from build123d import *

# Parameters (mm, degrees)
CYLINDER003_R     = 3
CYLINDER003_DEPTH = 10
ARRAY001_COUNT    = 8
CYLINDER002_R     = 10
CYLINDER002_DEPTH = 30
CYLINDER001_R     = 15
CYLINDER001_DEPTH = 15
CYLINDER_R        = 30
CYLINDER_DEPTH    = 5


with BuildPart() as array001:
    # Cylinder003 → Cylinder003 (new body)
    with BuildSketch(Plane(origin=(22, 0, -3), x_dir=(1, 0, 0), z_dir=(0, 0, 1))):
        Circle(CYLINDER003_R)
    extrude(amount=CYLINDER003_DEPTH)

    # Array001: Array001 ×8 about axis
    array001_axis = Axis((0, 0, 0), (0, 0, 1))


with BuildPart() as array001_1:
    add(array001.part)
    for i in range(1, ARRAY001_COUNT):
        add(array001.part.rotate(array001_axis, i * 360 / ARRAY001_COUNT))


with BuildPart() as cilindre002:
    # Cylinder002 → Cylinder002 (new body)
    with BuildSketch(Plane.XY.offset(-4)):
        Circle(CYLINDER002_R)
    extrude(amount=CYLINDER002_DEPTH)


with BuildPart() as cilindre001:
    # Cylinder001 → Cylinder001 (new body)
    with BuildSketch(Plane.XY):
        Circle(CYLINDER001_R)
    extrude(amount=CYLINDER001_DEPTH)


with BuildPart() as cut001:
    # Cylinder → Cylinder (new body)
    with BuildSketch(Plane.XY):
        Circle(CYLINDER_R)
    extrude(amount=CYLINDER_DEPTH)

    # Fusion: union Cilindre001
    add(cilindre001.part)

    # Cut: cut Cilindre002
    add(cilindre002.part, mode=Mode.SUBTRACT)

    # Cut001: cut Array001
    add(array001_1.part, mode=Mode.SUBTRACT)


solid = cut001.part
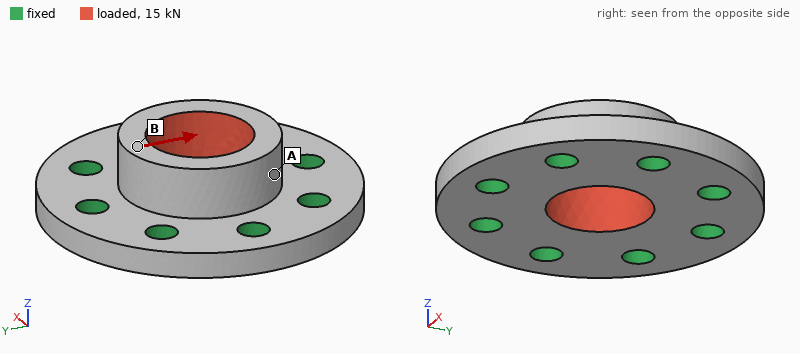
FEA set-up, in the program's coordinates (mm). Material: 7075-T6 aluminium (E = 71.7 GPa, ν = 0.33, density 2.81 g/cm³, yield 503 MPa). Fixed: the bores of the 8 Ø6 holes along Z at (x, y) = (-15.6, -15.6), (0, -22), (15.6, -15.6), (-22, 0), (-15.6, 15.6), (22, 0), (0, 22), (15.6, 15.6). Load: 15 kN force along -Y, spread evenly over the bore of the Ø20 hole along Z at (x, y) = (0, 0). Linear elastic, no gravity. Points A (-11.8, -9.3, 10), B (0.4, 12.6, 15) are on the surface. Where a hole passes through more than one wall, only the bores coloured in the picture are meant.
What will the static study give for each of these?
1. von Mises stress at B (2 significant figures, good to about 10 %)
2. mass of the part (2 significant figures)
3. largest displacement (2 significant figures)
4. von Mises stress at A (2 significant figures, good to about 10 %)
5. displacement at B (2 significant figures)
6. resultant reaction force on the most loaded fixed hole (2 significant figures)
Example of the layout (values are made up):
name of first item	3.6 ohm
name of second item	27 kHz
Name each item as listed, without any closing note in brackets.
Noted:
von Mises stress at B	48 MPa
mass of the part	43 g
largest displacement	25 µm
von Mises stress at A	19 MPa
displacement at B	24 µm
resultant reaction force on the most loaded fixed hole	3.0 kN
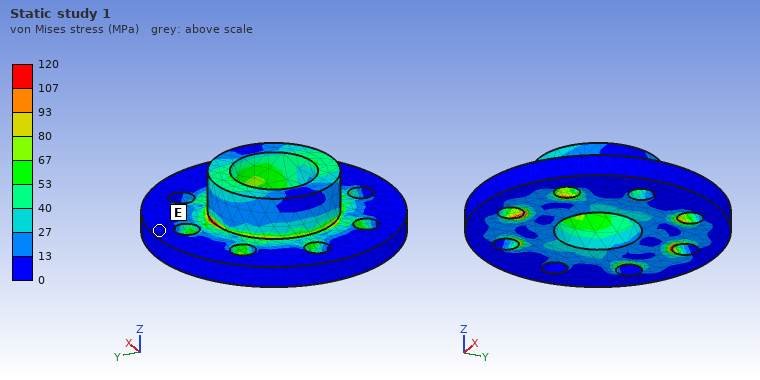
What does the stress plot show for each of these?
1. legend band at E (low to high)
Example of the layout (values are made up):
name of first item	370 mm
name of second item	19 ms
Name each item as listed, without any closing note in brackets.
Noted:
legend band at E	0 to 13 MPa
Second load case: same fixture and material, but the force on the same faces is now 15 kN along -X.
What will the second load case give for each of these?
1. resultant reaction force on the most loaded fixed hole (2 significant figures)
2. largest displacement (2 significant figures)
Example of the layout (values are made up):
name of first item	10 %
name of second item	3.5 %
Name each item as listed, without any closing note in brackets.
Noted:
resultant reaction force on the most loaded fixed hole	3.0 kN
largest displacement	25 µm
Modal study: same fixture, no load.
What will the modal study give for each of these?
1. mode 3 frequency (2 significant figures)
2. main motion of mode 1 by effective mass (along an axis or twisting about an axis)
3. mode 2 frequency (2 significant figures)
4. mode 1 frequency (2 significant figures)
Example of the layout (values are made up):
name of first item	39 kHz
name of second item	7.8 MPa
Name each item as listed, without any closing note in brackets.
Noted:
mode 3 frequency	36 kHz
main motion of mode 1 by effective mass	along Z
mode 2 frequency	36 kHz
mode 1 frequency	33 kHz
